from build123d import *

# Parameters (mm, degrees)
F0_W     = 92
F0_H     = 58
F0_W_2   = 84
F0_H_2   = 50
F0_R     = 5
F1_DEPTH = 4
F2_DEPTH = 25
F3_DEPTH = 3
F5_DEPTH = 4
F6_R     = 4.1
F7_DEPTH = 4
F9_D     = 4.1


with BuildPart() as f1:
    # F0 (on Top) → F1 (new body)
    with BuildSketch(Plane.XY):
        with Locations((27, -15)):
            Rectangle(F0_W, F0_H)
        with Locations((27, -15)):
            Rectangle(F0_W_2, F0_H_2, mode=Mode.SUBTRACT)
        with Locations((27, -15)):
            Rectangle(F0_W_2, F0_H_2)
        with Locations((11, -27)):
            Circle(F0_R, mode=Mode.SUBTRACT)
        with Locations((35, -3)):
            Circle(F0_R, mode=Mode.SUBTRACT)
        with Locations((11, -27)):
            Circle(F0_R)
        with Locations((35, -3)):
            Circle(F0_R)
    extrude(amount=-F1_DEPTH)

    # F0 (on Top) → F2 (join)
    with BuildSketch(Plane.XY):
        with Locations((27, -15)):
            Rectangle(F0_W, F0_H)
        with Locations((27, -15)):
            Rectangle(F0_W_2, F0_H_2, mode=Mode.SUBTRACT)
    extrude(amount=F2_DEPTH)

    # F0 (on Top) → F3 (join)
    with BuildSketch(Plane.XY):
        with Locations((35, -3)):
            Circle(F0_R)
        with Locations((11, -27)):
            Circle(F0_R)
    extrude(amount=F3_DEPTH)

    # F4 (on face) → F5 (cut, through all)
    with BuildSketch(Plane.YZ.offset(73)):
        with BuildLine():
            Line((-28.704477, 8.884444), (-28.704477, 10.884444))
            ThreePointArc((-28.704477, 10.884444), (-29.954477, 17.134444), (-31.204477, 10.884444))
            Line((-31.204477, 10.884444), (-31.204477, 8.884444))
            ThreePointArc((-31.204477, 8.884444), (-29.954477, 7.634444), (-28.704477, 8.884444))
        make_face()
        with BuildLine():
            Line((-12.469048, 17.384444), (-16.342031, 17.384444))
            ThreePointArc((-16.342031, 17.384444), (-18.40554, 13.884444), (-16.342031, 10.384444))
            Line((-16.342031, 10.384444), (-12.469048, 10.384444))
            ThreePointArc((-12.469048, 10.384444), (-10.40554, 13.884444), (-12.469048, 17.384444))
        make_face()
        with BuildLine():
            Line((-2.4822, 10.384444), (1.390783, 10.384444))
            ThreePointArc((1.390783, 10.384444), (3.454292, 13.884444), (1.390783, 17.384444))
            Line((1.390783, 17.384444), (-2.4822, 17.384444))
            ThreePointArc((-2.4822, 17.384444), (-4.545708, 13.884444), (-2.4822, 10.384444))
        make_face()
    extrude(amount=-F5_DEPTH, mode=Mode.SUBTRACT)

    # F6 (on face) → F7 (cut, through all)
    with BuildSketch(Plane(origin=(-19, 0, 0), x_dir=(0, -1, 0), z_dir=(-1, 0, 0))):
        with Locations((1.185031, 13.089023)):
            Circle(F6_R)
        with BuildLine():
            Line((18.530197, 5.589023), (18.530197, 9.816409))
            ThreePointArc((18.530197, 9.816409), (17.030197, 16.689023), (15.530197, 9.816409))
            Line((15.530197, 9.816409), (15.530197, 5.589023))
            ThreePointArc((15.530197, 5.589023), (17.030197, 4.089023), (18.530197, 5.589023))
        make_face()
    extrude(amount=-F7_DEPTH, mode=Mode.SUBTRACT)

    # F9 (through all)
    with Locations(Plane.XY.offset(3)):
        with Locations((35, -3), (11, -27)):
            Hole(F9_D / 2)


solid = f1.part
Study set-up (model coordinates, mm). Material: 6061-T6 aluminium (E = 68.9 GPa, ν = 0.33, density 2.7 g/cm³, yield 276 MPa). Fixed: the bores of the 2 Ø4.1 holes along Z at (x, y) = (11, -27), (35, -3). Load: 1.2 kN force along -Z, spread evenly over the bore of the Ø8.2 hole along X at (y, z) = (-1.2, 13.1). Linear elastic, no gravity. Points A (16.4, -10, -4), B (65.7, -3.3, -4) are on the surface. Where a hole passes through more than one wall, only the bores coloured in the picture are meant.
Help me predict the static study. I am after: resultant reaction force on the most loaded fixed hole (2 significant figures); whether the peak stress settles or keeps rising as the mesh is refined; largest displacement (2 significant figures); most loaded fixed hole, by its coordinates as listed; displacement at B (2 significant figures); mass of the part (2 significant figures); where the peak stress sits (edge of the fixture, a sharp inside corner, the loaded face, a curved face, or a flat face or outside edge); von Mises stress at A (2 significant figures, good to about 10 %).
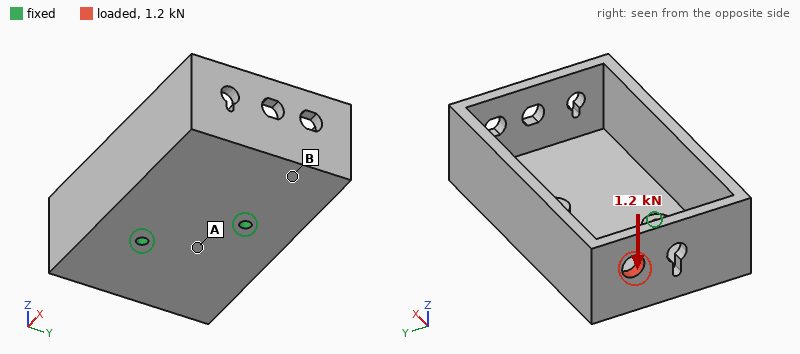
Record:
1000 N
keeps rising
0.64 mm
(11, -27)
0.21 mm
130 g
edge of the fixture
73 MPa
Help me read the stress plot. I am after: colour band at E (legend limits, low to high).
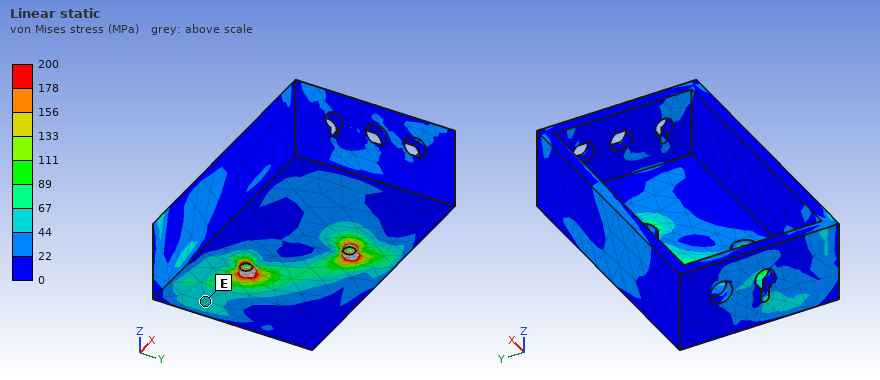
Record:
44 to 67 MPa
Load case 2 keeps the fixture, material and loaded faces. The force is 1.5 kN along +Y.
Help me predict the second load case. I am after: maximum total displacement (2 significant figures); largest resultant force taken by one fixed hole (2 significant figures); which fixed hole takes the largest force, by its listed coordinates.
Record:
0.32 mm
2.3 kN
(11, -27)
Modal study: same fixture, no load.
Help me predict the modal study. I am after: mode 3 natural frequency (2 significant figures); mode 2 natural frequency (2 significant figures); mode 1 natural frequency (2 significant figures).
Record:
2600 Hz
1700 Hz
1100 Hz
